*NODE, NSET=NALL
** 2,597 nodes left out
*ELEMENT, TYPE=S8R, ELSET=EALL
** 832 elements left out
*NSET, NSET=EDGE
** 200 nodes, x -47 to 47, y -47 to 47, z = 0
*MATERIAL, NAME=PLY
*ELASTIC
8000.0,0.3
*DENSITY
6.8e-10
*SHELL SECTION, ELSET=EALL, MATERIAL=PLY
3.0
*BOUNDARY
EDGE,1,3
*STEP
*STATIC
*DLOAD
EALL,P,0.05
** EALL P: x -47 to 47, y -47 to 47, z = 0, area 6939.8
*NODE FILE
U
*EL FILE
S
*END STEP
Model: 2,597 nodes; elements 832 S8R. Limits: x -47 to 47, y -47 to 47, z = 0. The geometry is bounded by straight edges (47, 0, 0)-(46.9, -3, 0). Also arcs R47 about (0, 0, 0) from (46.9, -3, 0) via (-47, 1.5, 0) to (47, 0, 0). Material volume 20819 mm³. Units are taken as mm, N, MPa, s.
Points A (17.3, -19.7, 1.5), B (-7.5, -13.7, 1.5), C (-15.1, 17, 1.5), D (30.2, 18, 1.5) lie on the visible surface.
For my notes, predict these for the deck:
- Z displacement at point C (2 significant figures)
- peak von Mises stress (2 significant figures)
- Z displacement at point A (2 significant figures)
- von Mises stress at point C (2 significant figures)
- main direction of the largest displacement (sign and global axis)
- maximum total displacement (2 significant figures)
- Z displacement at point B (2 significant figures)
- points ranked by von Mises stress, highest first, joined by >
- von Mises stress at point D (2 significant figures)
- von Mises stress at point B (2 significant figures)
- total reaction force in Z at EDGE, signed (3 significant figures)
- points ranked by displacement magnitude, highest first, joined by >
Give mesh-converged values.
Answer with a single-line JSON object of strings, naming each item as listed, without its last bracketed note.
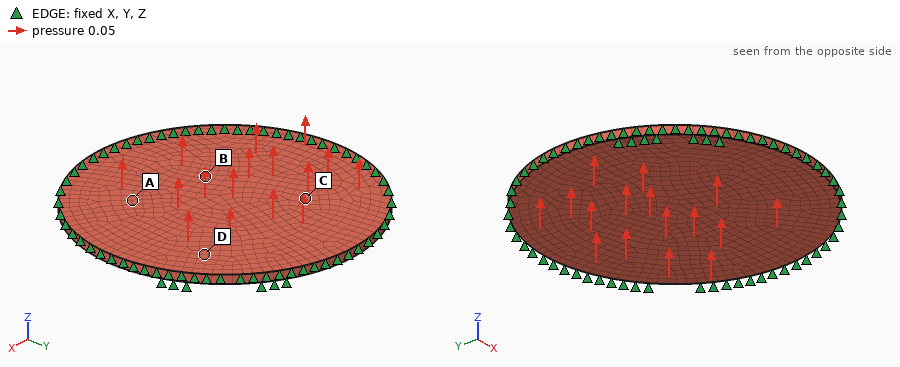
{"Z displacement at point C": "0.57 mm", "peak von Mises stress": "15 MPa", "Z displacement at point A": "0.50 mm", "von Mises stress at point C": "12 MPa", "main direction of the largest displacement": "+Z", "maximum total displacement": "0.79 mm", "Z displacement at point B": "0.68 mm", "points ranked by von Mises stress, highest first, joined by >": "B > C > A > D", "von Mises stress at point D": "9.1 MPa", "von Mises stress at point B": "14 MPa", "total reaction force in Z at EDGE, signed": "-347 N", "points ranked by displacement magnitude, highest first, joined by >": "B > C > A > D"}
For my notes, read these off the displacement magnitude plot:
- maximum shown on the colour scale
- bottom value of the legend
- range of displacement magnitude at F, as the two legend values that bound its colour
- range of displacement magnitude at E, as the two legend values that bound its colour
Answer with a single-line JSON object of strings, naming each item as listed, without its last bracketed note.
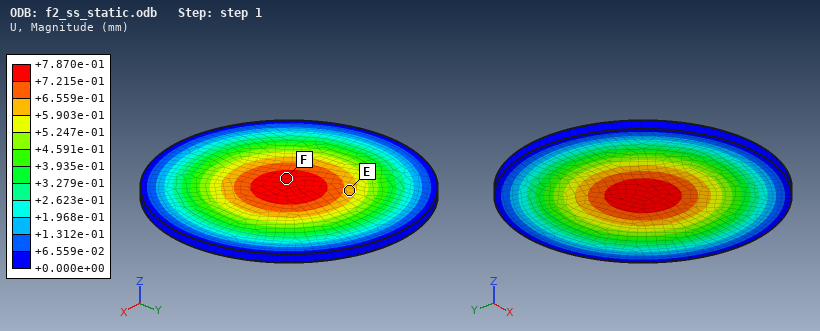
{"maximum shown on the colour scale": "+7.870e-01 mm", "bottom value of the legend": "+0.000e+00 mm", "range of displacement magnitude at F, as the two legend values that bound its colour": "+7.215e-01 to +7.870e-01 mm", "range of displacement magnitude at E, as the two legend values that bound its colour": "+5.903e-01 to +6.559e-01 mm"}
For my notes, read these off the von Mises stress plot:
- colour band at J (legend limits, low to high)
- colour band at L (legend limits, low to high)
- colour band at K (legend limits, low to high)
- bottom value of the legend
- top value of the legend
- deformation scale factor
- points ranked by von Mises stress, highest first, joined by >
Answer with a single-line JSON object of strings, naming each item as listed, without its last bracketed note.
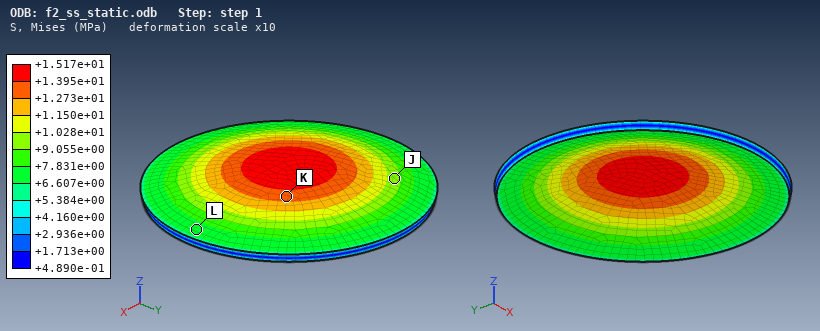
{"colour band at J": "+9.055e+00 to +1.028e+01 MPa", "colour band at L": "+6.607e+00 to +7.831e+00 MPa", "colour band at K": "+1.273e+01 to +1.395e+01 MPa", "bottom value of the legend": "+4.890e-01 MPa", "top value of the legend": "+1.517e+01 MPa", "deformation scale factor": "10", "points ranked by von Mises stress, highest first, joined by >": "K > J > L"}
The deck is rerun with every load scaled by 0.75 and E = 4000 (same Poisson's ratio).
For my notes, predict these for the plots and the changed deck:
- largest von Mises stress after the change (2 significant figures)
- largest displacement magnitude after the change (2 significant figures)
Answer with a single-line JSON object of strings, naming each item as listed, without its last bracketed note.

{"largest von Mises stress after the change": "11 MPa", "largest displacement magnitude after the change": "1.2 mm"}
